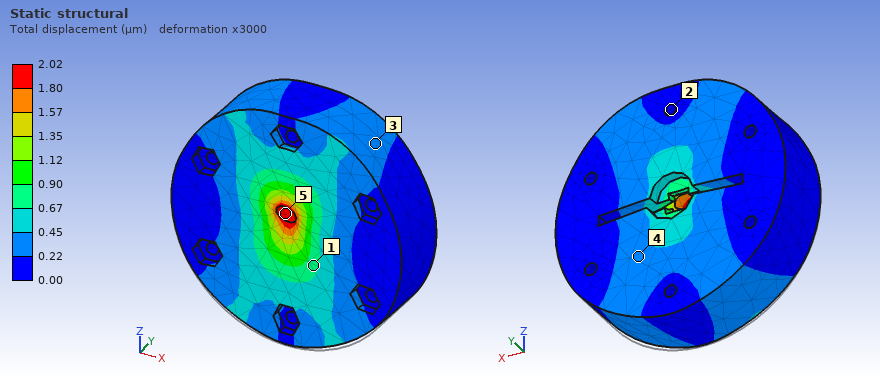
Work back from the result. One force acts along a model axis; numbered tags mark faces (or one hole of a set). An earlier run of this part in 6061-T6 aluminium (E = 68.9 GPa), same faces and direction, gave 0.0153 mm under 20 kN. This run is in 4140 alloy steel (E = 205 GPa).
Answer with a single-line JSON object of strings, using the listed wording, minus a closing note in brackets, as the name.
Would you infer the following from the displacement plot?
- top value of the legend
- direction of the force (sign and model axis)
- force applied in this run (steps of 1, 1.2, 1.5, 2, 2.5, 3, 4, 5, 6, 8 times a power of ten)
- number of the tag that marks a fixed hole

{"top value of the legend": "2.02 µm", "direction of the force": "+Z", "force applied in this run": "8 kN", "number of the tag that marks a fixed hole": "2"}
